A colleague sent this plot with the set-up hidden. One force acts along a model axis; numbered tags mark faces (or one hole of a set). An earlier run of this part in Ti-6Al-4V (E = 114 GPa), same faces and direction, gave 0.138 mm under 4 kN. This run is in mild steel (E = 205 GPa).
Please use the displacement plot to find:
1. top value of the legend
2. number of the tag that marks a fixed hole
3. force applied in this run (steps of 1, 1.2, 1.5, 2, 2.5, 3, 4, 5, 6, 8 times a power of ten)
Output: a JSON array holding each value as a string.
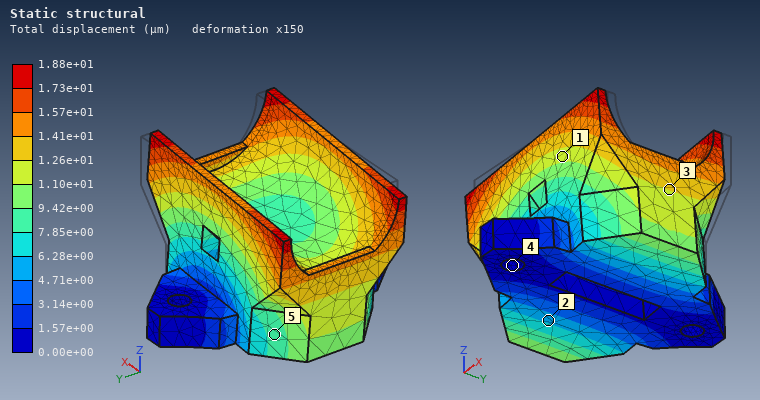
["1.88e+01 µm", "4", "1 kN"]
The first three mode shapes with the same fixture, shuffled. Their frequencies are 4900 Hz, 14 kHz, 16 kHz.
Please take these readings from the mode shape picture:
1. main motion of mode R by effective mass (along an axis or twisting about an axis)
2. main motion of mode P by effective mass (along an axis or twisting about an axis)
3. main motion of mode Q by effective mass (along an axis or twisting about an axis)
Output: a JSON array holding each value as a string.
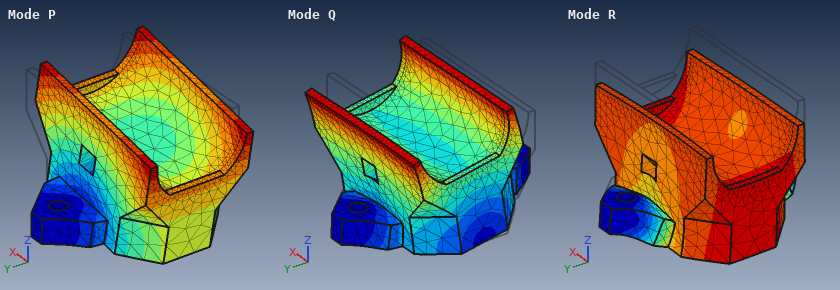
["along Z", "along X", "along Y"]
